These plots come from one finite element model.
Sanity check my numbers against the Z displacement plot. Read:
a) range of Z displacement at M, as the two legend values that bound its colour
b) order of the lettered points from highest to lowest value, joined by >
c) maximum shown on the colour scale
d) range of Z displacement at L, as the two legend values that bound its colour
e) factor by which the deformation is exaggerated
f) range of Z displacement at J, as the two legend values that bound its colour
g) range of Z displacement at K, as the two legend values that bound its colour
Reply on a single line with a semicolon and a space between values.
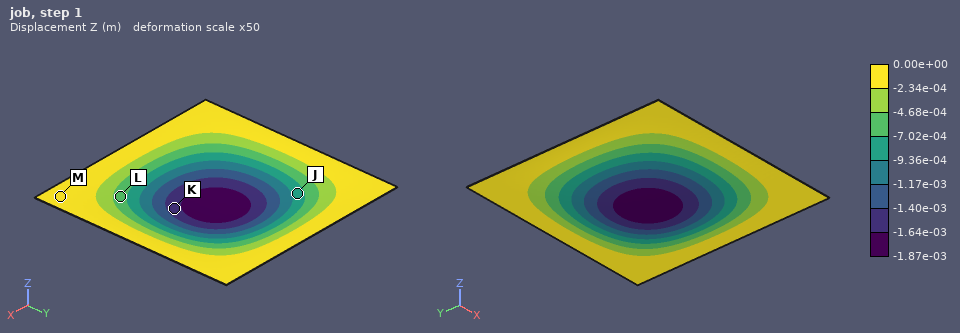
-2.34e-04 to 0.00e+00 m; M > L > J > K; 0.00e+00 m; -7.02e-04 to -4.68e-04 m; 50; -9.36e-04 to -7.02e-04 m; -1.64e-03 to -1.40e-03 m
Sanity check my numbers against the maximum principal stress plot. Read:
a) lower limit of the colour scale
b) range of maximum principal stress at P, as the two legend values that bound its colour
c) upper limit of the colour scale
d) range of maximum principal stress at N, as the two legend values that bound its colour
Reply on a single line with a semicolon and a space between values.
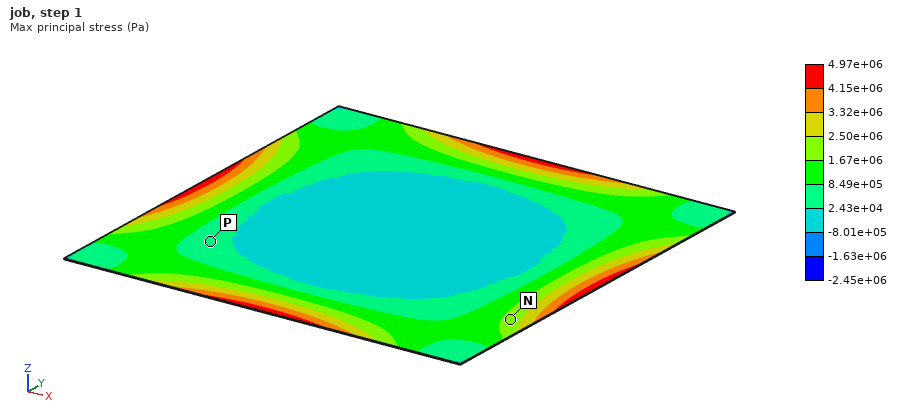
-2.45e+06 Pa; 2.43e+04 to 8.49e+05 Pa; 4.97e+06 Pa; 1.67e+06 to 2.50e+06 Pa
